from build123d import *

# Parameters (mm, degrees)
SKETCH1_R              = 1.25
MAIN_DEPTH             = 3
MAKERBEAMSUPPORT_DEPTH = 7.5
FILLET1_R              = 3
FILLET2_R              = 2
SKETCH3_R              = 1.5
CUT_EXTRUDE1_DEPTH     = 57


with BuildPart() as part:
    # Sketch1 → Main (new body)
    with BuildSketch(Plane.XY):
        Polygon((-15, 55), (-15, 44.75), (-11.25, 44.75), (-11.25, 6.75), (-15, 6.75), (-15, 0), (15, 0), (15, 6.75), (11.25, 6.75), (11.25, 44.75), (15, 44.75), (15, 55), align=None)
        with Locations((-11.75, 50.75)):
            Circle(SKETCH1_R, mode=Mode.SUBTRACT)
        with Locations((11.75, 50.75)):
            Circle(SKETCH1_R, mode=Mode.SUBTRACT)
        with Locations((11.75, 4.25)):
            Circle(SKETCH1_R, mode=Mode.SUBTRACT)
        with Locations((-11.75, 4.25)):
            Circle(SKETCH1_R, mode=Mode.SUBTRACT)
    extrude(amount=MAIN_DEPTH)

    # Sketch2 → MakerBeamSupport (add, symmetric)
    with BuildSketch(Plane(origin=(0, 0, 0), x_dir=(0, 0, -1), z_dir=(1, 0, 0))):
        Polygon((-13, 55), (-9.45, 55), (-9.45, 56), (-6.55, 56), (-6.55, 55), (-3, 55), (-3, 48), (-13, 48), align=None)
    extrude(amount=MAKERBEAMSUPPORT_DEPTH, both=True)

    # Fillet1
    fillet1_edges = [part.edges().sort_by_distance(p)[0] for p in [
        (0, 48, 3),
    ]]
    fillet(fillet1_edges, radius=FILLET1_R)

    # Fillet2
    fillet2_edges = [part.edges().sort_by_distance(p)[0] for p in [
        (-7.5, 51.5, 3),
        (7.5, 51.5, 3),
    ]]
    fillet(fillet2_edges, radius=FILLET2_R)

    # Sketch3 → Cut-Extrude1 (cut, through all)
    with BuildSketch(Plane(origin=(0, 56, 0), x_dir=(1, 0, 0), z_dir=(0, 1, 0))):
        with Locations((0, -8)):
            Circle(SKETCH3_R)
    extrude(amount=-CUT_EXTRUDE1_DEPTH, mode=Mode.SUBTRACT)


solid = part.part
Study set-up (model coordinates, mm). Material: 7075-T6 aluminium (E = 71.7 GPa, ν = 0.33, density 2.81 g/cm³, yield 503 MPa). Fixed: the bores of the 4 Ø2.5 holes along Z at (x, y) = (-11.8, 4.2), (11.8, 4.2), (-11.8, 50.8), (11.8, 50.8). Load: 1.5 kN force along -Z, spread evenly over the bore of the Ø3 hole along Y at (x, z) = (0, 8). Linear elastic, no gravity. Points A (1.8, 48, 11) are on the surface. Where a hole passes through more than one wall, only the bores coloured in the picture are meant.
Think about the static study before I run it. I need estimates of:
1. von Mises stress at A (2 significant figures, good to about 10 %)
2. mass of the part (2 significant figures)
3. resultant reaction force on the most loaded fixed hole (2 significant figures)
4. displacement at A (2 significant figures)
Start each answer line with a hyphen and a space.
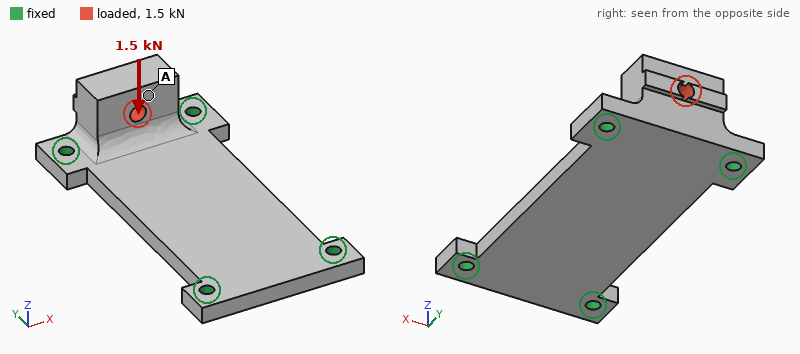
- 20 MPa
- 14 g
- 870 N
- 18 µm
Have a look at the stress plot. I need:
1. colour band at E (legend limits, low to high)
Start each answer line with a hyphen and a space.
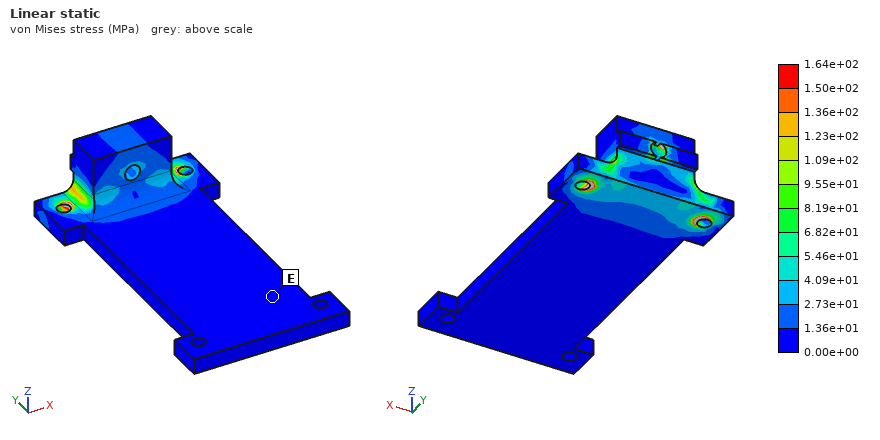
- 0.00e+00 to 1.36e+01 MPa
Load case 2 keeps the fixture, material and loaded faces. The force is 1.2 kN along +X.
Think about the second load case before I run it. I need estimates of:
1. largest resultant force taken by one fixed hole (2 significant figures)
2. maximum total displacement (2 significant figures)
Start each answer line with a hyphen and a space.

- 710 N
- 11 µm
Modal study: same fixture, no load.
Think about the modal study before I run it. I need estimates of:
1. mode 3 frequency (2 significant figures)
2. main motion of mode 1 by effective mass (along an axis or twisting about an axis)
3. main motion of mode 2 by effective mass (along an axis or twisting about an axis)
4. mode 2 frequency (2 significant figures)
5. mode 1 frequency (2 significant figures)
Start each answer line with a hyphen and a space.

- 14 kHz
- along Z
- twisting about Y
- 12 kHz
- 6200 Hz
